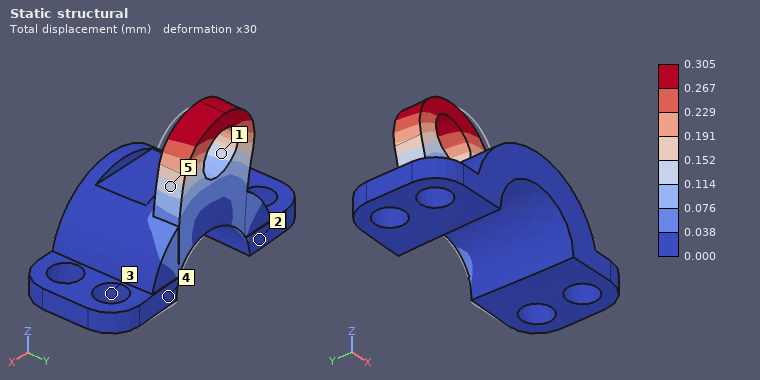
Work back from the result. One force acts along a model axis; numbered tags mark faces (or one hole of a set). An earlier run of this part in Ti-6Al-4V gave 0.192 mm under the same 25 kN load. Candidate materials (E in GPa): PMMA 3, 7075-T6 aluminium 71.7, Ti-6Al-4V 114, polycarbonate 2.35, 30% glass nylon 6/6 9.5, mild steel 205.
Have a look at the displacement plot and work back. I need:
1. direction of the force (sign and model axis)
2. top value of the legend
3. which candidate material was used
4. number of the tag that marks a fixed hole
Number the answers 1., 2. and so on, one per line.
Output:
1. -X
2. 0.305 mm
3. 7075-T6 aluminium
4. 3
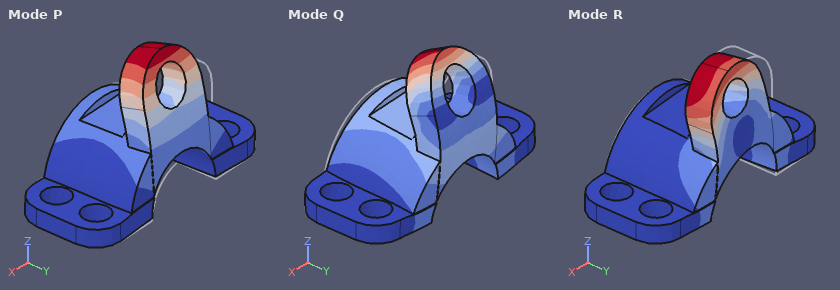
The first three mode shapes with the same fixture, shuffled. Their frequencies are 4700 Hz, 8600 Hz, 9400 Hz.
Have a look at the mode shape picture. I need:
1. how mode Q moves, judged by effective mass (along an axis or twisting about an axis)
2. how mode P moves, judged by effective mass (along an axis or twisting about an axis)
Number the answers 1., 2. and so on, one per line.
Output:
1. along Y
2. along Y
